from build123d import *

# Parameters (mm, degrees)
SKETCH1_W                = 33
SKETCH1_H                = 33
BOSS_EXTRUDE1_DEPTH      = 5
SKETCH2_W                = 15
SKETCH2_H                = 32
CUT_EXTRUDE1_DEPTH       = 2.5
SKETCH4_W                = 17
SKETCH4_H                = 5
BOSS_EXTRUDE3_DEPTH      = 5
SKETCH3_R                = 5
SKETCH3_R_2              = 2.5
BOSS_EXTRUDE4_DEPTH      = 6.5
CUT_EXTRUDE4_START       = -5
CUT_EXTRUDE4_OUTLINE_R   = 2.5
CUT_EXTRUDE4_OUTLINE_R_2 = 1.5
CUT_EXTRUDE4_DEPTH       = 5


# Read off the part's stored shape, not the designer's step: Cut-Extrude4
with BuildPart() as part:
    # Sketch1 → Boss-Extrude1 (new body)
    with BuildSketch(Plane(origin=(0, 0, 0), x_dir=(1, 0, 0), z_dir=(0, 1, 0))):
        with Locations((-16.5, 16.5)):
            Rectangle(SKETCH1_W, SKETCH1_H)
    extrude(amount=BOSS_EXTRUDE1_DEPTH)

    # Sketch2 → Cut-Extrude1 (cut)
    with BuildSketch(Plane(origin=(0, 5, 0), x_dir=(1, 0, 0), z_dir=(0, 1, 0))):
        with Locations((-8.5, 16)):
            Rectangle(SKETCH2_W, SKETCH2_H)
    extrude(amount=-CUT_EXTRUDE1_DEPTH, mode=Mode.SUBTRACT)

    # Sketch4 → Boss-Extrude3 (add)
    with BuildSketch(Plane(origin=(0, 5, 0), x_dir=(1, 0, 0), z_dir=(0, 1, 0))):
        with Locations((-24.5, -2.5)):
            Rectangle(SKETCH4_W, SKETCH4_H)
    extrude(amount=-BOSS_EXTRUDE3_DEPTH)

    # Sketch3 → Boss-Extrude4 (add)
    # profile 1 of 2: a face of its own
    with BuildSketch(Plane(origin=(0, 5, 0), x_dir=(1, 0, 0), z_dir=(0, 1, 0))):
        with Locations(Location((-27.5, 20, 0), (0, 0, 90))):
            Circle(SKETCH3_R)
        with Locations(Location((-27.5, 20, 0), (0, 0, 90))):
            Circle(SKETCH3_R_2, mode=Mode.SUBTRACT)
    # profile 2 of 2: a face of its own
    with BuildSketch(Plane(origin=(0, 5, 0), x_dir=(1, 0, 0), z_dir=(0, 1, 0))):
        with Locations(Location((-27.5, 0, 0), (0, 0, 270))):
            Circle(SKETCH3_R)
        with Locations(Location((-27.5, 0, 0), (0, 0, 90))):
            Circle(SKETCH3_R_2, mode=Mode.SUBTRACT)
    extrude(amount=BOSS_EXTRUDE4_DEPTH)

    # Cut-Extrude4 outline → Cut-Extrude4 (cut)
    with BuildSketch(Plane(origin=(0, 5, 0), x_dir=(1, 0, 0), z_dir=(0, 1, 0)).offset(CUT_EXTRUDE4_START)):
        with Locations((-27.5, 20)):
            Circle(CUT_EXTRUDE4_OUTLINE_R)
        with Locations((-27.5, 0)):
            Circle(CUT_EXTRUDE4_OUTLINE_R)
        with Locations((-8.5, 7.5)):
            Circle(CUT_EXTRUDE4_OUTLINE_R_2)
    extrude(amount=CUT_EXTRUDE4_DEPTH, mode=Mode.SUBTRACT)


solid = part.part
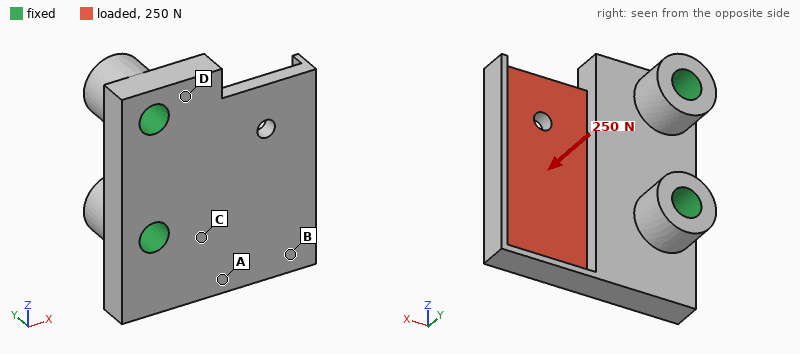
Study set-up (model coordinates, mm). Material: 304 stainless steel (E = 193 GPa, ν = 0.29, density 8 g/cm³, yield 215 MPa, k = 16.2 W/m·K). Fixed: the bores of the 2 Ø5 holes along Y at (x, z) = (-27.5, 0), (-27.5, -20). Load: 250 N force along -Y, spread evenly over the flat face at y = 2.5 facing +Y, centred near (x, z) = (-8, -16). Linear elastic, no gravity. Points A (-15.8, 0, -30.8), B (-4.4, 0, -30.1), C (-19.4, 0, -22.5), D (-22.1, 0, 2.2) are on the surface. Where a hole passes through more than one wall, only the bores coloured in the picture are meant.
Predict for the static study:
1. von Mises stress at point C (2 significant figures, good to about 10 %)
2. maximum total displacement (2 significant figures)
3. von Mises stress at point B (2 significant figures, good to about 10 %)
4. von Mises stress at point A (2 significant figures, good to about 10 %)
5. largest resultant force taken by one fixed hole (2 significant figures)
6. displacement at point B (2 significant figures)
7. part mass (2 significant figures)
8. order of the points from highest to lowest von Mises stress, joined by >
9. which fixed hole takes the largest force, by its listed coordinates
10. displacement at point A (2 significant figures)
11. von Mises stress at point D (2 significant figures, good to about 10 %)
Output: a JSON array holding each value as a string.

["22 MPa", "26 µm", "5.9 MPa", "31 MPa", "190 N", "17 µm", "42 g", "A > C > D > B", "(-27.5, -20)", "4.2 µm", "15 MPa"]
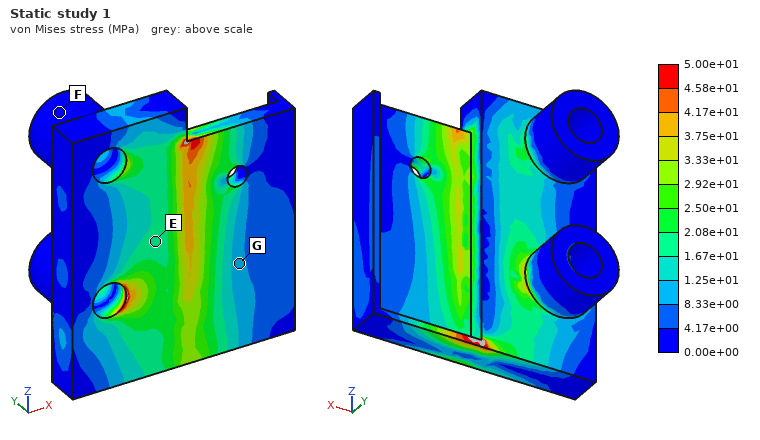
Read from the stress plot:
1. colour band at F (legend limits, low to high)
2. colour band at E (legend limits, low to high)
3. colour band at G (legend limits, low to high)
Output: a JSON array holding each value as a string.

["0.00e+00 to 4.17e+00 MPa", "1.67e+01 to 2.08e+01 MPa", "8.33e+00 to 1.25e+01 MPa"]
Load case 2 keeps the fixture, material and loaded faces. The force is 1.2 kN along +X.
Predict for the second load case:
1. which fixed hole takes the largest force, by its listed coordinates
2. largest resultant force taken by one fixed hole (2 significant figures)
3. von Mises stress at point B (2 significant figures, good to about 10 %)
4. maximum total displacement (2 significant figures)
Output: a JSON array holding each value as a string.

["(-27.5, -20)", "900 N", "8.9 MPa", "17 µm"]
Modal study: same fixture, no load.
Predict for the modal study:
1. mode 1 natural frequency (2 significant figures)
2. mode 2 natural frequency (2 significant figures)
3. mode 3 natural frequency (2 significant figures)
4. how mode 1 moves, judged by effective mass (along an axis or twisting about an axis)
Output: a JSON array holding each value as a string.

["5300 Hz", "8300 Hz", "19 kHz", "along Y"]
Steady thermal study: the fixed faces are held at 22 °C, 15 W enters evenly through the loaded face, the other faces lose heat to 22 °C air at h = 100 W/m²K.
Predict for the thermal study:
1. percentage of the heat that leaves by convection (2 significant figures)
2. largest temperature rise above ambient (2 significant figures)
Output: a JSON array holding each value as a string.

["54 %", "77 K"]
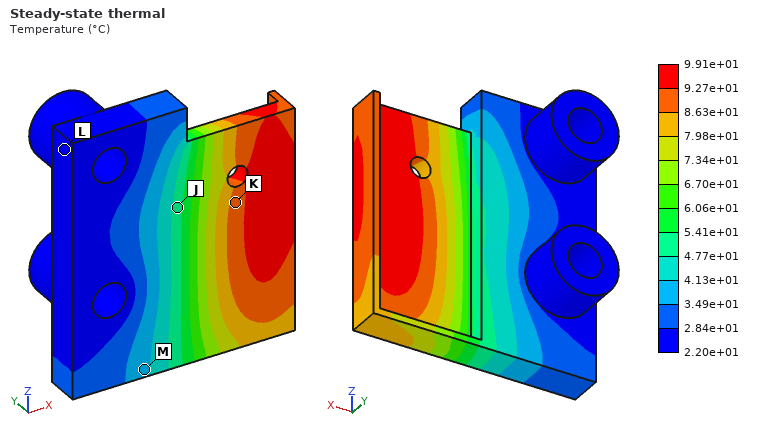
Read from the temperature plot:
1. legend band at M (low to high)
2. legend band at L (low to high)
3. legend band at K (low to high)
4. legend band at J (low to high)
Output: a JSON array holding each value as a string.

["3.49e+01 to 4.13e+01 °C", "2.20e+01 to 2.84e+01 °C", "8.63e+01 to 9.27e+01 °C", "4.77e+01 to 5.41e+01 °C"]
